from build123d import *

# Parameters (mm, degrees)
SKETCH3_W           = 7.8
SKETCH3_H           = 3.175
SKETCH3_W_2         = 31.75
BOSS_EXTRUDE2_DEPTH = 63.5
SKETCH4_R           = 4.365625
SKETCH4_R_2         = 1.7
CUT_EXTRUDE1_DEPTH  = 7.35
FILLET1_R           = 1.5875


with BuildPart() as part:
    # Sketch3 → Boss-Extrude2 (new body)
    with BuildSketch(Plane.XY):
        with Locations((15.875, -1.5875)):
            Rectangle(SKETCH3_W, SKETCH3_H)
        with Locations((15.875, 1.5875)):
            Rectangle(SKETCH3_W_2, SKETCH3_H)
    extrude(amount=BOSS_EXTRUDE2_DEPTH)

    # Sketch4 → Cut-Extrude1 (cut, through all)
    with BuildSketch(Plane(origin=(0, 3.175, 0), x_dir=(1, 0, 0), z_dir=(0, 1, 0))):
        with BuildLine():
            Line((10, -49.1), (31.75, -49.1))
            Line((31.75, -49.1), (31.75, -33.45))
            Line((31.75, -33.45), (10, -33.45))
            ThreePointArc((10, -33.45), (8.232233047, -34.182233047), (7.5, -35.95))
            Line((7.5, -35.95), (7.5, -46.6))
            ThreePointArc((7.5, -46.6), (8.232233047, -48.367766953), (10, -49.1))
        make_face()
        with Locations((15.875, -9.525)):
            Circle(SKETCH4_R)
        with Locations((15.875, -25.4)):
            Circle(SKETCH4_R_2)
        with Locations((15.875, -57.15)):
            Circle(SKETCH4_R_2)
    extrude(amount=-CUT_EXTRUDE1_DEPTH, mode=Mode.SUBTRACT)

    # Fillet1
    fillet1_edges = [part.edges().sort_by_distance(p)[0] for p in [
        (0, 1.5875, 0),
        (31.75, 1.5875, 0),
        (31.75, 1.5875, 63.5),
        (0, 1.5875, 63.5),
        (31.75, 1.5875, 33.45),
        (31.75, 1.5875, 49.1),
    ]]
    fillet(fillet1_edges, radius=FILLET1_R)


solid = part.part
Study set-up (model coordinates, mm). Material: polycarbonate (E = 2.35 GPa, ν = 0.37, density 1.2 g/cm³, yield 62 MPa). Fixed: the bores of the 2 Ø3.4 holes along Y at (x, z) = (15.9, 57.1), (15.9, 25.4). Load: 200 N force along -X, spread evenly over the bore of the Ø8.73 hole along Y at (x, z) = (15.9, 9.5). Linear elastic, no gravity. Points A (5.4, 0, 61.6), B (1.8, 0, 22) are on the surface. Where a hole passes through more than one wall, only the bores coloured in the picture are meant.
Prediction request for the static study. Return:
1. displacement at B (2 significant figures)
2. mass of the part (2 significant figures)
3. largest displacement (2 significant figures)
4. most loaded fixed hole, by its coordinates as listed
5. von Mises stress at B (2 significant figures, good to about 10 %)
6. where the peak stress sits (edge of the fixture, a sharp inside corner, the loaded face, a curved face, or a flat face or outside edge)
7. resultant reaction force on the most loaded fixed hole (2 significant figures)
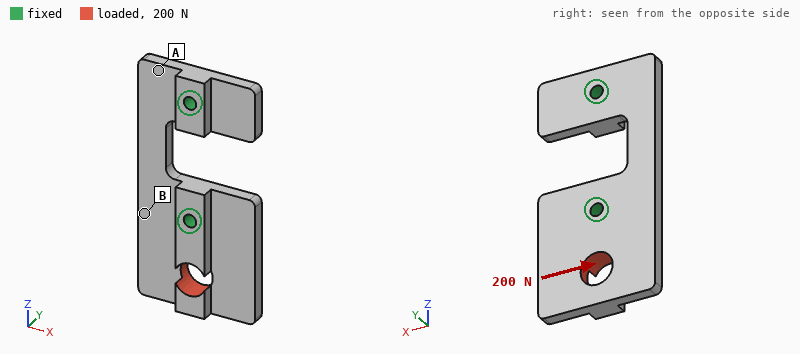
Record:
0.11 mm
7.1 g
0.34 mm
(15.9, 25.4)
5.6 MPa
edge of the fixture
250 N
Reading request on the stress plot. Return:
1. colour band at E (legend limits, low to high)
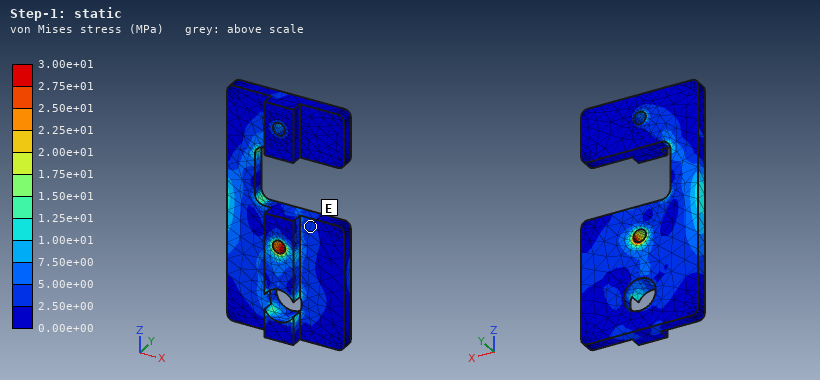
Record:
2.50e+00 to 5.00e+00 MPa
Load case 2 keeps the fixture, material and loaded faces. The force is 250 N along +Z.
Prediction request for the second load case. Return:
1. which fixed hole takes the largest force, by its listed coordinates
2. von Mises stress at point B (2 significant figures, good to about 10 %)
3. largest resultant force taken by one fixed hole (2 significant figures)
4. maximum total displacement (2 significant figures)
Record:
(15.9, 25.4)
1.6 MPa
240 N
0.23 mm
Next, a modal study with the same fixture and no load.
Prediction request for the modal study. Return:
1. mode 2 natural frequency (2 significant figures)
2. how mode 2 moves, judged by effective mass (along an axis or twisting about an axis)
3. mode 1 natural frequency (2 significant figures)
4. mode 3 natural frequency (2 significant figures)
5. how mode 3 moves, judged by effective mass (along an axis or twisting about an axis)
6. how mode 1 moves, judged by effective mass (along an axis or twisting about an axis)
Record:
1900 Hz
twisting about Z
1400 Hz
2700 Hz
along X
along Y
